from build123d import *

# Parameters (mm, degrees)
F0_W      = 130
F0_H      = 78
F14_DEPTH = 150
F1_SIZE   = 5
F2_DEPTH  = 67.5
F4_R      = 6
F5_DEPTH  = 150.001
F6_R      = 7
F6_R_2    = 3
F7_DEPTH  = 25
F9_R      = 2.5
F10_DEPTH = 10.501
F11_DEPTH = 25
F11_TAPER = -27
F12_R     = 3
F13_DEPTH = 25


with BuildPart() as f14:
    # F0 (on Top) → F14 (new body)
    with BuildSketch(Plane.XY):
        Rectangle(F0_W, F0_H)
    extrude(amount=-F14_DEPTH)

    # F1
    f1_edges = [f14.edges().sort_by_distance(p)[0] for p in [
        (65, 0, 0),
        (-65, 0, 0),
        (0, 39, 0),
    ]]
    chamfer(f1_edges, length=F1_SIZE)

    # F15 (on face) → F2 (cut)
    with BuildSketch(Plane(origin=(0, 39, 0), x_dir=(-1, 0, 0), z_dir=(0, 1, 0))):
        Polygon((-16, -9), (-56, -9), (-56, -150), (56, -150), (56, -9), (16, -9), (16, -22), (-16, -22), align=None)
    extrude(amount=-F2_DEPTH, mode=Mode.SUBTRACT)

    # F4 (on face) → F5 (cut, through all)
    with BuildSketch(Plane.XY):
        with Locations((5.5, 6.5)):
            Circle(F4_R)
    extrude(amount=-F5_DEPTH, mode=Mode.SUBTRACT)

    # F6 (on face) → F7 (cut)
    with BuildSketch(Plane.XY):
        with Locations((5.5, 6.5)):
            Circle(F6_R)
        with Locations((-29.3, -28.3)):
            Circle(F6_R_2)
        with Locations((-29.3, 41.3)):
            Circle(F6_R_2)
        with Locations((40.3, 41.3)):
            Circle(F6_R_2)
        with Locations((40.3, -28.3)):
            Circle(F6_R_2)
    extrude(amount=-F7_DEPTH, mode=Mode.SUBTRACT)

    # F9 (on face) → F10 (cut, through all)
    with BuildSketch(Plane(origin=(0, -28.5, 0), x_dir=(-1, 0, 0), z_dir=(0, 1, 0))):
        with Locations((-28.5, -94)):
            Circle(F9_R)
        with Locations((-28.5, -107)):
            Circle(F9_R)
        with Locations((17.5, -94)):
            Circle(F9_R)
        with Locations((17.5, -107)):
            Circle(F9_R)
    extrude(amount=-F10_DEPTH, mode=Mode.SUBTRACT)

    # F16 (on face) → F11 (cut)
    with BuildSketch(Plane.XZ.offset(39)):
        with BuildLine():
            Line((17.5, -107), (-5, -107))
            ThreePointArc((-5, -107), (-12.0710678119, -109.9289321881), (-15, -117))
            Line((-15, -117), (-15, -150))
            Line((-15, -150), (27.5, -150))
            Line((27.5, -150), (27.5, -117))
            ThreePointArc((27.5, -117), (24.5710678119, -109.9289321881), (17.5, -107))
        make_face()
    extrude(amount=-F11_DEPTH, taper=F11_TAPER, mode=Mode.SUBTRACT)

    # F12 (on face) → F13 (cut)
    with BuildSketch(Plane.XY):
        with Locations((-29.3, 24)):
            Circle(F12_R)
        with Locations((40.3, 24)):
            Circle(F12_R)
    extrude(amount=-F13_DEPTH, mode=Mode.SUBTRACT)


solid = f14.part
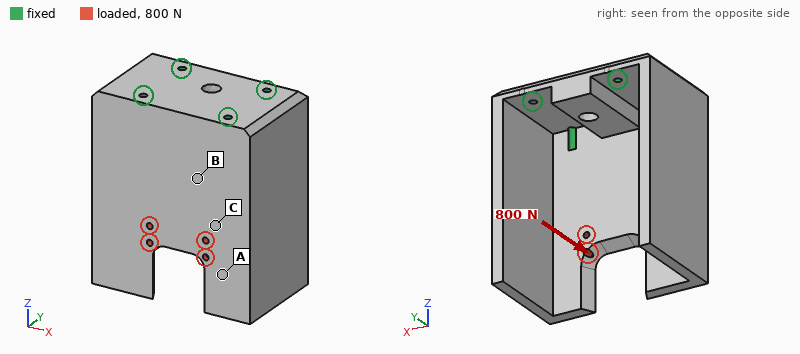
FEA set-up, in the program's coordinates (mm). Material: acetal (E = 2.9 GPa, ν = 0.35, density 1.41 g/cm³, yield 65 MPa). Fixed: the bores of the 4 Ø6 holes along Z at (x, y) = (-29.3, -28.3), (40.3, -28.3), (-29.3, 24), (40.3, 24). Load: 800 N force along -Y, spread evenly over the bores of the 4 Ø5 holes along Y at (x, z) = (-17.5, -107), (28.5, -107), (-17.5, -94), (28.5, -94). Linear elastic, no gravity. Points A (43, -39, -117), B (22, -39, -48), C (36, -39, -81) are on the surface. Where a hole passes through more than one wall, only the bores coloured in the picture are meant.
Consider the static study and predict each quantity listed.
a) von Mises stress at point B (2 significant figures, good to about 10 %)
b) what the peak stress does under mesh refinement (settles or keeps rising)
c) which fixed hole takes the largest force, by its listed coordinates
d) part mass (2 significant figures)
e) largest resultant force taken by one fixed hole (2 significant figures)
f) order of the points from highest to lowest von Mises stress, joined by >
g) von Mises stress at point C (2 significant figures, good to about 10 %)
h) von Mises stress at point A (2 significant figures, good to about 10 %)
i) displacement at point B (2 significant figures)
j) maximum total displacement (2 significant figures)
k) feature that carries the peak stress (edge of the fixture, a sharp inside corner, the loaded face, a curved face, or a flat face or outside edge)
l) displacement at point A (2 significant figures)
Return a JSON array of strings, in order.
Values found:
["4.0 MPa", "keeps rising", "(40.3, -28.3)", "640 g", "640 N", "C > B > A", "7.0 MPa", "1.7 MPa", "0.27 mm", "1.7 mm", "a sharp inside corner", "0.84 mm"]
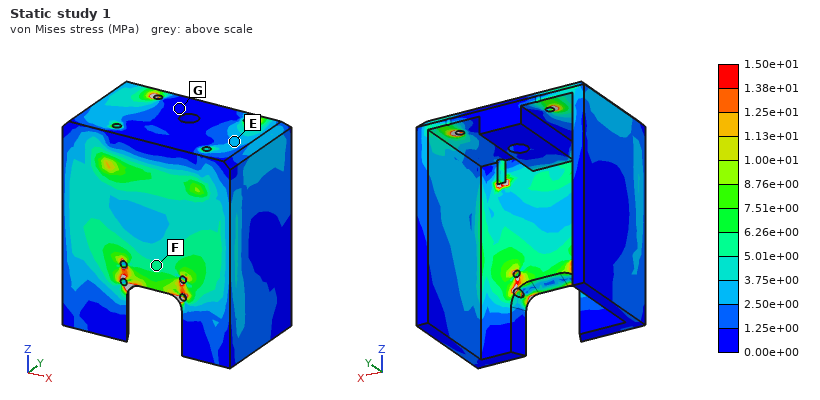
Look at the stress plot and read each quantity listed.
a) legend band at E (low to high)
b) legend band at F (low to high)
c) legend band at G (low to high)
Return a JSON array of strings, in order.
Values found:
["2.50e+00 to 3.75e+00 MPa", "5.01e+00 to 6.26e+00 MPa", "0.00e+00 to 1.25e+00 MPa"]
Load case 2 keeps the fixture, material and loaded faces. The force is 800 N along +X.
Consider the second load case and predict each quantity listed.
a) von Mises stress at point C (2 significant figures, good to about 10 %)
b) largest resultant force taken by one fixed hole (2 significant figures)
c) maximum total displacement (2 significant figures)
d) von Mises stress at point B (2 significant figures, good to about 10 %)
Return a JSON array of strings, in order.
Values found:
["0.98 MPa", "880 N", "0.24 mm", "1.7 MPa"]
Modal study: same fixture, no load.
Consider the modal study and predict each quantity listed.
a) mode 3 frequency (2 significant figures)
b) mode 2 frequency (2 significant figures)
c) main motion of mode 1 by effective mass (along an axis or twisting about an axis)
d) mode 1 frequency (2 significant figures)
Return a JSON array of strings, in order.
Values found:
["340 Hz", "310 Hz", "along Y", "270 Hz"]
